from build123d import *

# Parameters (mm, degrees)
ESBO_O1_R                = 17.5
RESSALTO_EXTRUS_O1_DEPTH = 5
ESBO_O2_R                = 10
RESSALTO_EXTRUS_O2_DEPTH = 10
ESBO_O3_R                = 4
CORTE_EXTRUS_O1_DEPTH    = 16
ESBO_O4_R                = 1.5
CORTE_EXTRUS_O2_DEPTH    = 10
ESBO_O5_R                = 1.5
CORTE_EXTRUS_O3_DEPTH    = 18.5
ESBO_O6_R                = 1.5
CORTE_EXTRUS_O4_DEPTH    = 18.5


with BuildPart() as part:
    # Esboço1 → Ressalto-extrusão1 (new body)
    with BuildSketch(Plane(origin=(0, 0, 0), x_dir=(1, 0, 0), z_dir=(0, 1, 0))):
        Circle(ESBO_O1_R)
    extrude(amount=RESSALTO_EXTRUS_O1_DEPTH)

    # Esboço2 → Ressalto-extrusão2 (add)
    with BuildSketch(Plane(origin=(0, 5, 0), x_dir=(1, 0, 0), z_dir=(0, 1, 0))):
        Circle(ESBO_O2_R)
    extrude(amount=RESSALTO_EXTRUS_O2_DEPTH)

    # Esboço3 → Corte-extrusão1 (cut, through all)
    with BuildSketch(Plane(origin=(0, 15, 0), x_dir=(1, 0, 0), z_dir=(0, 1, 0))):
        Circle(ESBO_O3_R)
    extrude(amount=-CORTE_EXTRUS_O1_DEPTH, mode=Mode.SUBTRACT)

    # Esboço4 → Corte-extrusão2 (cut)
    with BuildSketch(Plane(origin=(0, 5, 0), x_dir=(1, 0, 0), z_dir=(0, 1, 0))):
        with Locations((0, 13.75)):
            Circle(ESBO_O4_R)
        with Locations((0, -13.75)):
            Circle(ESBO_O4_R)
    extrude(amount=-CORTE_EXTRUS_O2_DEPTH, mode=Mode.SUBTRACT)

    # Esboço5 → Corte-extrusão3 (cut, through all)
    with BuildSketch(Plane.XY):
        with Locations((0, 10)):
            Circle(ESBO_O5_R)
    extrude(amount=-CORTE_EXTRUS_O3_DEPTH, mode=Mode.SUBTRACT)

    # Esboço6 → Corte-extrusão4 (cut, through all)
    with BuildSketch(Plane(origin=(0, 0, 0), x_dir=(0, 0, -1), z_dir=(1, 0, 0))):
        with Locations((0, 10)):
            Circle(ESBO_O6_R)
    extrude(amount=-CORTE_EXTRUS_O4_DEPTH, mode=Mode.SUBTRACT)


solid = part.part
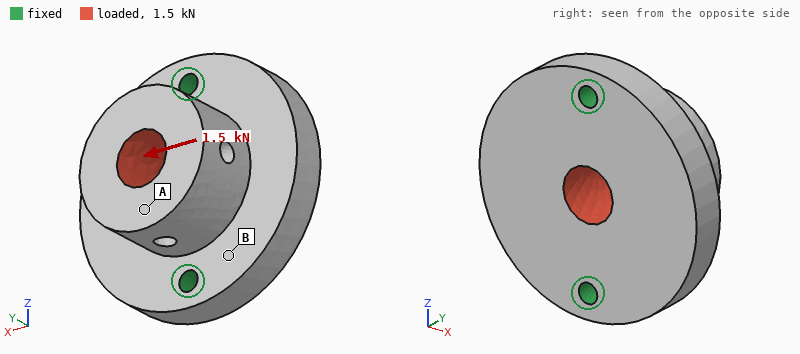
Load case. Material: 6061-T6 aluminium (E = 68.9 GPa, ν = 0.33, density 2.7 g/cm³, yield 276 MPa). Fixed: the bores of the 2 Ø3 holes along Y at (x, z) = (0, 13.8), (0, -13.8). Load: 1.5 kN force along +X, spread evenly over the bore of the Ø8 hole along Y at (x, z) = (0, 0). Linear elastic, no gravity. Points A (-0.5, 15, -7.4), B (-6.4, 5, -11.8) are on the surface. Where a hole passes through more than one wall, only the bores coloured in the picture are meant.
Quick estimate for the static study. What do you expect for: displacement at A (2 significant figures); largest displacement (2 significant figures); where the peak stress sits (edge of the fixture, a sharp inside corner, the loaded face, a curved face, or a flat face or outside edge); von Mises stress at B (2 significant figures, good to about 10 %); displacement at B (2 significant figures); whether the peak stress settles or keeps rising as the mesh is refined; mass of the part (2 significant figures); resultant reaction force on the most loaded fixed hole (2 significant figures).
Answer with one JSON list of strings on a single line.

["21 µm", "26 µm", "edge of the fixture", "25 MPa", "7.5 µm", "keeps rising", "19 g", "750 N"]
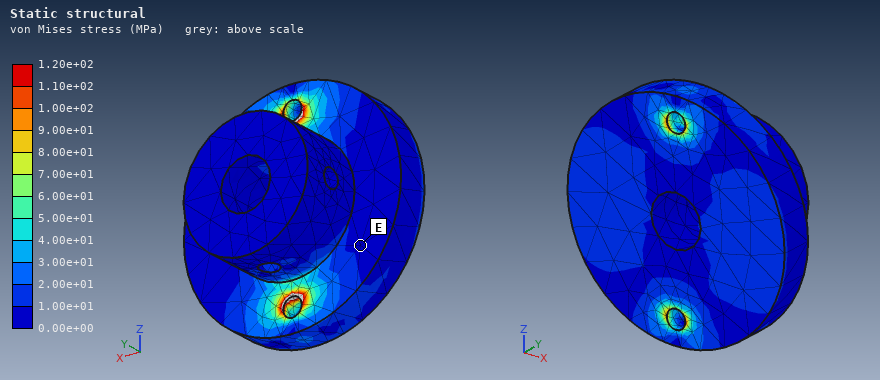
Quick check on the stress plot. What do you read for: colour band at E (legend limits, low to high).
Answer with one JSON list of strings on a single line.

["0.00e+00 to 1.00e+01 MPa"]
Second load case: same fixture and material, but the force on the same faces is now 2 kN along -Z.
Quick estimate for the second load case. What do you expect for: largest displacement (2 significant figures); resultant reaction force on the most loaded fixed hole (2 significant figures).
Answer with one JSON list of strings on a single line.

["6.6 µm", "1.1 kN"]
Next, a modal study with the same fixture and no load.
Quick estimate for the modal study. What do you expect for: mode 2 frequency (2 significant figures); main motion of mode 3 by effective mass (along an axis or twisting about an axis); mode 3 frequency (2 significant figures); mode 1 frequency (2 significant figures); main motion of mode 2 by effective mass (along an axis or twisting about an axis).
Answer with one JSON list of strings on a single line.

["18 kHz", "along Z", "28 kHz", "9000 Hz", "along Y"]
